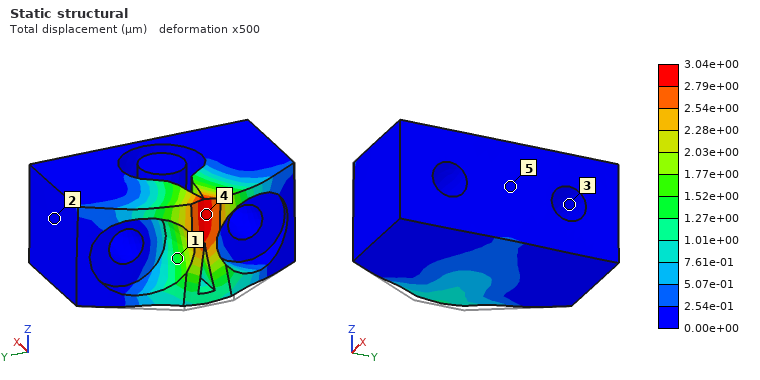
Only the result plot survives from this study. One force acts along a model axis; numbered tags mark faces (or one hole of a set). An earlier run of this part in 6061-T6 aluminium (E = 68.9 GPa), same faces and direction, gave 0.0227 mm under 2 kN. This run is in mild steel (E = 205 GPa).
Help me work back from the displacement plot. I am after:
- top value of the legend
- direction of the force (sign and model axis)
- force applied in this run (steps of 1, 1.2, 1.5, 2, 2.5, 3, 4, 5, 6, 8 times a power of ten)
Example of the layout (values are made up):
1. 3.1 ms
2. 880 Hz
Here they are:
1. 3.04e+00 µm
2. +X
3. 800 N
